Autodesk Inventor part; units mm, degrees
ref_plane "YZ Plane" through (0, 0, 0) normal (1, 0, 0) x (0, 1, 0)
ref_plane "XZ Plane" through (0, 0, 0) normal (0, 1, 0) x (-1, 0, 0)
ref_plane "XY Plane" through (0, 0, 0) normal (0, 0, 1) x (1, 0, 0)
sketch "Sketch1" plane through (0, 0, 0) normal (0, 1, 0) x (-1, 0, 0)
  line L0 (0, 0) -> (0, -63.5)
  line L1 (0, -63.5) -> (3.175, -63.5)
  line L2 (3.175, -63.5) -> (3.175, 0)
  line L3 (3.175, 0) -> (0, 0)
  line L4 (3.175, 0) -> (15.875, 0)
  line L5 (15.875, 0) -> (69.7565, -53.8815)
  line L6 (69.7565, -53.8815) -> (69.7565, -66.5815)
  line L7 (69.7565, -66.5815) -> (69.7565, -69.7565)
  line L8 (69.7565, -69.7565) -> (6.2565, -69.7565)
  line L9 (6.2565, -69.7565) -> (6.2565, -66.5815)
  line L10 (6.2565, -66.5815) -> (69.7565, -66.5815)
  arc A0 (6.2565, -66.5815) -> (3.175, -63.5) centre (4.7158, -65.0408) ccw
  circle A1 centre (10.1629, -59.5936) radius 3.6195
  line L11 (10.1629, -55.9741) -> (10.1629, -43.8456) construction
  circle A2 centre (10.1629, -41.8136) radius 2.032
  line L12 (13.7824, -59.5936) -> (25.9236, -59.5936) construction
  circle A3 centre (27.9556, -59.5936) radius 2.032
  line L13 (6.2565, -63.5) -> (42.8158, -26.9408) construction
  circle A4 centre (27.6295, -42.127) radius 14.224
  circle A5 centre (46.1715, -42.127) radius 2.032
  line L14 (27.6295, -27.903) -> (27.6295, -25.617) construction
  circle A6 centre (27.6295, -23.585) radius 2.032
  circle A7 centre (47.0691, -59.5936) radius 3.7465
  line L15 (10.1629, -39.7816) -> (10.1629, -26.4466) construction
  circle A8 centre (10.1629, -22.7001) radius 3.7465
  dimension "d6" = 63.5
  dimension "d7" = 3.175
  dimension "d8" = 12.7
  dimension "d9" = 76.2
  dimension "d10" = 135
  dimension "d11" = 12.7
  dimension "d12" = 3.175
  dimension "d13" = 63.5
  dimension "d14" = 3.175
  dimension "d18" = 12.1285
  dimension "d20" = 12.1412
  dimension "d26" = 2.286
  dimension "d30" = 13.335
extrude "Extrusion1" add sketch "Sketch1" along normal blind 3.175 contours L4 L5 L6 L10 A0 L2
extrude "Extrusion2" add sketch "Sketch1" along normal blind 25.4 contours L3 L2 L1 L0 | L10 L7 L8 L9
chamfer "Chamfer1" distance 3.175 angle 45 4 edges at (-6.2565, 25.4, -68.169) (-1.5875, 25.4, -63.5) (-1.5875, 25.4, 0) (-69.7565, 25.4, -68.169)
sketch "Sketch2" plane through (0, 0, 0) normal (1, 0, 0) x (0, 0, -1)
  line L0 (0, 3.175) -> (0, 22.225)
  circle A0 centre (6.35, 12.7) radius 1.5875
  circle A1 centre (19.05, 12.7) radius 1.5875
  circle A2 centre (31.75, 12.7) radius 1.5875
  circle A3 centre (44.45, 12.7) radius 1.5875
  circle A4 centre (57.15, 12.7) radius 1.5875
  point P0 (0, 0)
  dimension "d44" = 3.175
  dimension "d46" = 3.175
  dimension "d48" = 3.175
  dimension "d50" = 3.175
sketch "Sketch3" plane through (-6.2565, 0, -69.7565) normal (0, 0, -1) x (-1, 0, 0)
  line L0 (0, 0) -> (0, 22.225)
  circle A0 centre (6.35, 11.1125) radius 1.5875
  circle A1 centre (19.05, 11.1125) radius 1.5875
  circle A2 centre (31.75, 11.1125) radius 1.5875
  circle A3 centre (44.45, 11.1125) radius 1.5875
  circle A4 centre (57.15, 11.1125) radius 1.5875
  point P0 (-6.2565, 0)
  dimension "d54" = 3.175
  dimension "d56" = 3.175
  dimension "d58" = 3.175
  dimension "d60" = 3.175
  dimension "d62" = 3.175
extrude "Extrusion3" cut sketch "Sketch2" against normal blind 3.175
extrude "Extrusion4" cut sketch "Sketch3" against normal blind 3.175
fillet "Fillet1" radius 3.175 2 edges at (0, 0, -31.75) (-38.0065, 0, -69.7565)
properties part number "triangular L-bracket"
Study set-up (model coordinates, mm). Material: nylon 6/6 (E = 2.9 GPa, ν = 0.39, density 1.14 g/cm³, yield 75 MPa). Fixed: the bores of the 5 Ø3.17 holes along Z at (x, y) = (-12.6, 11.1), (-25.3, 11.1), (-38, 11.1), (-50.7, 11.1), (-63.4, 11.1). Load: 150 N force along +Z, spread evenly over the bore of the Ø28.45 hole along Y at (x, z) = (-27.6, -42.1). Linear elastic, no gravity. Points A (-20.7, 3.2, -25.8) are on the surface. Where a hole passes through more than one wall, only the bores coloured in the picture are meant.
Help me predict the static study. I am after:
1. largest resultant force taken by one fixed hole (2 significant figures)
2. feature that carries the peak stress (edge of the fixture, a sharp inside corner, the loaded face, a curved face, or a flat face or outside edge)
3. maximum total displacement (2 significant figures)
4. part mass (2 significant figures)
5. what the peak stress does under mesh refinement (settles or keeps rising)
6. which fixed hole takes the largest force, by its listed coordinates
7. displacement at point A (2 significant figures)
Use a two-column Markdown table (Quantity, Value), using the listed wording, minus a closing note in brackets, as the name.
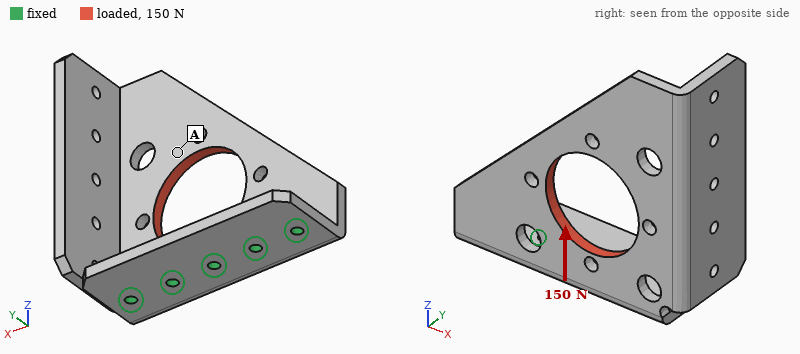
| Quantity | Value |
|---|---|
| largest resultant force taken by one fixed hole | 57 N |
| feature that carries the peak stress | edge of the fixture |
| maximum total displacement | 1.1 mm |
| part mass | 19 g |
| what the peak stress does under mesh refinement | keeps rising |
| which fixed hole takes the largest force, by its listed coordinates | (-12.6, 11.1) |
| displacement at point A | 0.63 mm |
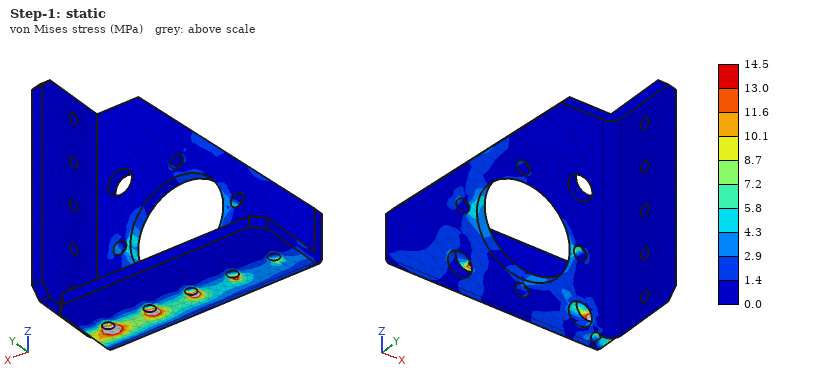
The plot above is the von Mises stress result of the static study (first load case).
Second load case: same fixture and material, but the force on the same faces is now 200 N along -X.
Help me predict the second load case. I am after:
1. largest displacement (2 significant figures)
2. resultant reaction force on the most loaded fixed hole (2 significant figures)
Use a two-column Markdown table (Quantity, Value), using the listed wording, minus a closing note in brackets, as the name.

| Quantity | Value |
|---|---|
| largest displacement | 1.1 mm |
| resultant reaction force on the most loaded fixed hole | 96 N |
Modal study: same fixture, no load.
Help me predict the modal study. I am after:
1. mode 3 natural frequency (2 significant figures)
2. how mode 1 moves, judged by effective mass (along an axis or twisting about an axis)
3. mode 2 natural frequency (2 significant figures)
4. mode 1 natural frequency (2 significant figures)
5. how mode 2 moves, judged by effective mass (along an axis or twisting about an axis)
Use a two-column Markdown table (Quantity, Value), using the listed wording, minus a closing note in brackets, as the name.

| Quantity | Value |
|---|---|
| mode 3 natural frequency | 750 Hz |
| how mode 1 moves, judged by effective mass | along Y |
| mode 2 natural frequency | 390 Hz |
| mode 1 natural frequency | 120 Hz |
| how mode 2 moves, judged by effective mass | along X |
